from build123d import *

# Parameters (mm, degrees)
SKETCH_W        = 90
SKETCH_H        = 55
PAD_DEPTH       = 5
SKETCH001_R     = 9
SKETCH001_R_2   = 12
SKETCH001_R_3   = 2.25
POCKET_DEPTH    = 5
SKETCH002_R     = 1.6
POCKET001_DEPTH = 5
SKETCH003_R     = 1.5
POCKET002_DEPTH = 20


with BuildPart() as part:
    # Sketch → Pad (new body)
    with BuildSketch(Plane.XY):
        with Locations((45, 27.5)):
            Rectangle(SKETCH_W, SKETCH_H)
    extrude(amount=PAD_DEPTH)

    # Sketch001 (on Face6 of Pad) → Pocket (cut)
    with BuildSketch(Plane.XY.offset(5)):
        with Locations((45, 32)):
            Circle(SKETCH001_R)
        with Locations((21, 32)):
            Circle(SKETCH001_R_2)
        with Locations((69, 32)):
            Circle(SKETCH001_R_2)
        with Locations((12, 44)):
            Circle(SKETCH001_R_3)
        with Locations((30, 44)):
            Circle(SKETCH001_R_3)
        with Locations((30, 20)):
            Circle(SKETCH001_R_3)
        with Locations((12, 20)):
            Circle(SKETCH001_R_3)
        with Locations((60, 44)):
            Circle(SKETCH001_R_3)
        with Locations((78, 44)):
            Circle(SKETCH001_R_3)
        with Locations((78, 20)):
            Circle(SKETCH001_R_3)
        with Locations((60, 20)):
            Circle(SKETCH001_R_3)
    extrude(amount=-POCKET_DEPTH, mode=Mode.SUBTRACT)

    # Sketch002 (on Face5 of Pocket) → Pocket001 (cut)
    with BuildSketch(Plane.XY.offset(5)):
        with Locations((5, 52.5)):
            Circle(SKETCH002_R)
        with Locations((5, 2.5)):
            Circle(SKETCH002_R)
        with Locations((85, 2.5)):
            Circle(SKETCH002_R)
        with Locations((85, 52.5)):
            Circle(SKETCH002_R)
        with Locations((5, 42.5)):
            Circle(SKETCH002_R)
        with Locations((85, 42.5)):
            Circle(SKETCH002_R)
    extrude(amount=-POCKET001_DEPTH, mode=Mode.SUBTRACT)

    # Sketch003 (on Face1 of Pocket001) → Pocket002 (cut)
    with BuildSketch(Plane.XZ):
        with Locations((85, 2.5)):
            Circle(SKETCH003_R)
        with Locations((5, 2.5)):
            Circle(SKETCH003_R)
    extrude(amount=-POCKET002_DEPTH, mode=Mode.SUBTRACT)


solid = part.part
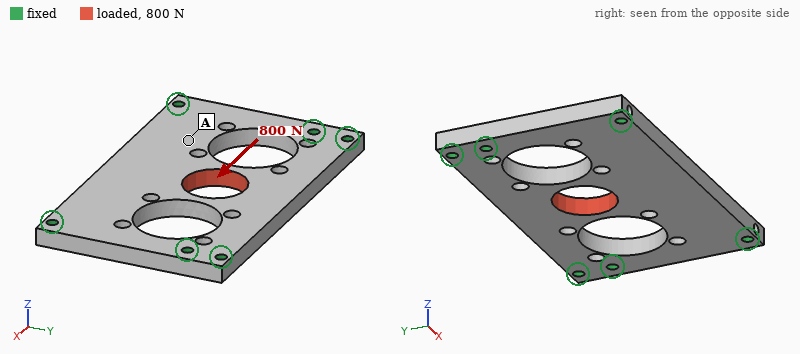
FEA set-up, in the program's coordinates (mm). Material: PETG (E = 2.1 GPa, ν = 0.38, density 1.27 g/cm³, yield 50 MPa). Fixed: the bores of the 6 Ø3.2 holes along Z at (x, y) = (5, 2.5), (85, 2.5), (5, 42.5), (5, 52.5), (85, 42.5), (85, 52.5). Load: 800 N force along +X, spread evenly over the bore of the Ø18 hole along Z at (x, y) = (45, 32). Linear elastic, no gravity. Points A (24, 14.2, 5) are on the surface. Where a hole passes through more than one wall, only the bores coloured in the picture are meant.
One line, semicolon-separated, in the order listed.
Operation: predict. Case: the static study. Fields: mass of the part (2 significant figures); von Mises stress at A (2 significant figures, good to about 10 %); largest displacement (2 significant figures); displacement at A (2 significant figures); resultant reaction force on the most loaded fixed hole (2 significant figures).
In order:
23 g; 2.7 MPa; 0.15 mm; 0.039 mm; 210 N
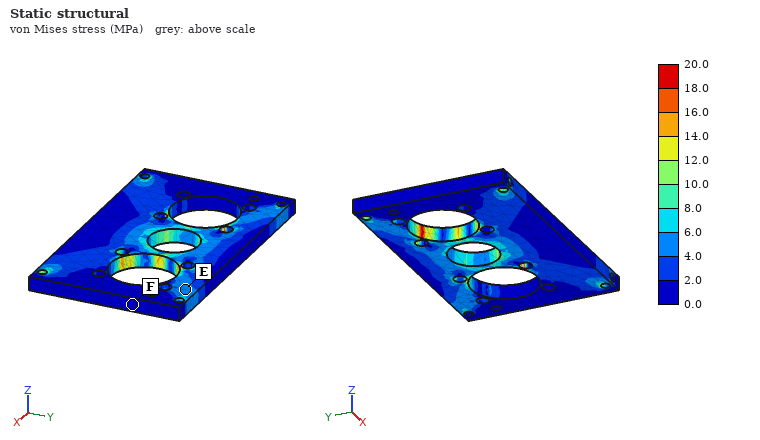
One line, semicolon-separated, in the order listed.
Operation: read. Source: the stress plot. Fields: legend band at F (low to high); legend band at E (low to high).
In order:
0.0 to 2.0 MPa; 4.0 to 6.0 MPa
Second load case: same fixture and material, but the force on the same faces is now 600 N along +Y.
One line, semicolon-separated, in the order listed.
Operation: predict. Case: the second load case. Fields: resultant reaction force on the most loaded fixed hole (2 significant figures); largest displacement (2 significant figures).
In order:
240 N; 0.25 mm
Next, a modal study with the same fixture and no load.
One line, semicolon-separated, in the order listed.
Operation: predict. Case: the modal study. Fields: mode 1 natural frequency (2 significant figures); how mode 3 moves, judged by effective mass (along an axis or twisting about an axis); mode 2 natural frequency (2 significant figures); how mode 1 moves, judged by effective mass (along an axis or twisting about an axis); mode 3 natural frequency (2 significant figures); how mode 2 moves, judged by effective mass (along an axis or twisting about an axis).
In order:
850 Hz; twisting about Y; 1200 Hz; along Z; 2200 Hz; twisting about X
